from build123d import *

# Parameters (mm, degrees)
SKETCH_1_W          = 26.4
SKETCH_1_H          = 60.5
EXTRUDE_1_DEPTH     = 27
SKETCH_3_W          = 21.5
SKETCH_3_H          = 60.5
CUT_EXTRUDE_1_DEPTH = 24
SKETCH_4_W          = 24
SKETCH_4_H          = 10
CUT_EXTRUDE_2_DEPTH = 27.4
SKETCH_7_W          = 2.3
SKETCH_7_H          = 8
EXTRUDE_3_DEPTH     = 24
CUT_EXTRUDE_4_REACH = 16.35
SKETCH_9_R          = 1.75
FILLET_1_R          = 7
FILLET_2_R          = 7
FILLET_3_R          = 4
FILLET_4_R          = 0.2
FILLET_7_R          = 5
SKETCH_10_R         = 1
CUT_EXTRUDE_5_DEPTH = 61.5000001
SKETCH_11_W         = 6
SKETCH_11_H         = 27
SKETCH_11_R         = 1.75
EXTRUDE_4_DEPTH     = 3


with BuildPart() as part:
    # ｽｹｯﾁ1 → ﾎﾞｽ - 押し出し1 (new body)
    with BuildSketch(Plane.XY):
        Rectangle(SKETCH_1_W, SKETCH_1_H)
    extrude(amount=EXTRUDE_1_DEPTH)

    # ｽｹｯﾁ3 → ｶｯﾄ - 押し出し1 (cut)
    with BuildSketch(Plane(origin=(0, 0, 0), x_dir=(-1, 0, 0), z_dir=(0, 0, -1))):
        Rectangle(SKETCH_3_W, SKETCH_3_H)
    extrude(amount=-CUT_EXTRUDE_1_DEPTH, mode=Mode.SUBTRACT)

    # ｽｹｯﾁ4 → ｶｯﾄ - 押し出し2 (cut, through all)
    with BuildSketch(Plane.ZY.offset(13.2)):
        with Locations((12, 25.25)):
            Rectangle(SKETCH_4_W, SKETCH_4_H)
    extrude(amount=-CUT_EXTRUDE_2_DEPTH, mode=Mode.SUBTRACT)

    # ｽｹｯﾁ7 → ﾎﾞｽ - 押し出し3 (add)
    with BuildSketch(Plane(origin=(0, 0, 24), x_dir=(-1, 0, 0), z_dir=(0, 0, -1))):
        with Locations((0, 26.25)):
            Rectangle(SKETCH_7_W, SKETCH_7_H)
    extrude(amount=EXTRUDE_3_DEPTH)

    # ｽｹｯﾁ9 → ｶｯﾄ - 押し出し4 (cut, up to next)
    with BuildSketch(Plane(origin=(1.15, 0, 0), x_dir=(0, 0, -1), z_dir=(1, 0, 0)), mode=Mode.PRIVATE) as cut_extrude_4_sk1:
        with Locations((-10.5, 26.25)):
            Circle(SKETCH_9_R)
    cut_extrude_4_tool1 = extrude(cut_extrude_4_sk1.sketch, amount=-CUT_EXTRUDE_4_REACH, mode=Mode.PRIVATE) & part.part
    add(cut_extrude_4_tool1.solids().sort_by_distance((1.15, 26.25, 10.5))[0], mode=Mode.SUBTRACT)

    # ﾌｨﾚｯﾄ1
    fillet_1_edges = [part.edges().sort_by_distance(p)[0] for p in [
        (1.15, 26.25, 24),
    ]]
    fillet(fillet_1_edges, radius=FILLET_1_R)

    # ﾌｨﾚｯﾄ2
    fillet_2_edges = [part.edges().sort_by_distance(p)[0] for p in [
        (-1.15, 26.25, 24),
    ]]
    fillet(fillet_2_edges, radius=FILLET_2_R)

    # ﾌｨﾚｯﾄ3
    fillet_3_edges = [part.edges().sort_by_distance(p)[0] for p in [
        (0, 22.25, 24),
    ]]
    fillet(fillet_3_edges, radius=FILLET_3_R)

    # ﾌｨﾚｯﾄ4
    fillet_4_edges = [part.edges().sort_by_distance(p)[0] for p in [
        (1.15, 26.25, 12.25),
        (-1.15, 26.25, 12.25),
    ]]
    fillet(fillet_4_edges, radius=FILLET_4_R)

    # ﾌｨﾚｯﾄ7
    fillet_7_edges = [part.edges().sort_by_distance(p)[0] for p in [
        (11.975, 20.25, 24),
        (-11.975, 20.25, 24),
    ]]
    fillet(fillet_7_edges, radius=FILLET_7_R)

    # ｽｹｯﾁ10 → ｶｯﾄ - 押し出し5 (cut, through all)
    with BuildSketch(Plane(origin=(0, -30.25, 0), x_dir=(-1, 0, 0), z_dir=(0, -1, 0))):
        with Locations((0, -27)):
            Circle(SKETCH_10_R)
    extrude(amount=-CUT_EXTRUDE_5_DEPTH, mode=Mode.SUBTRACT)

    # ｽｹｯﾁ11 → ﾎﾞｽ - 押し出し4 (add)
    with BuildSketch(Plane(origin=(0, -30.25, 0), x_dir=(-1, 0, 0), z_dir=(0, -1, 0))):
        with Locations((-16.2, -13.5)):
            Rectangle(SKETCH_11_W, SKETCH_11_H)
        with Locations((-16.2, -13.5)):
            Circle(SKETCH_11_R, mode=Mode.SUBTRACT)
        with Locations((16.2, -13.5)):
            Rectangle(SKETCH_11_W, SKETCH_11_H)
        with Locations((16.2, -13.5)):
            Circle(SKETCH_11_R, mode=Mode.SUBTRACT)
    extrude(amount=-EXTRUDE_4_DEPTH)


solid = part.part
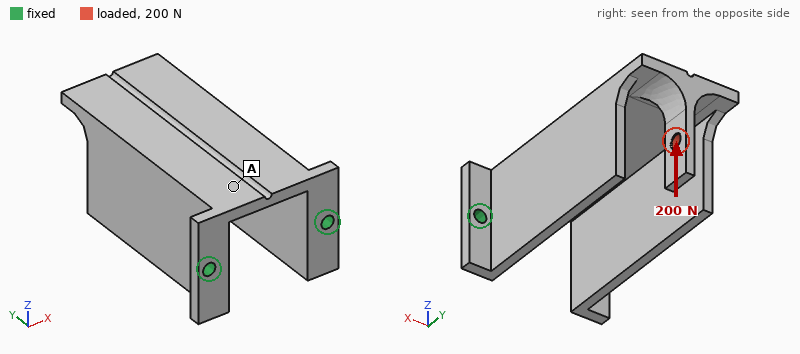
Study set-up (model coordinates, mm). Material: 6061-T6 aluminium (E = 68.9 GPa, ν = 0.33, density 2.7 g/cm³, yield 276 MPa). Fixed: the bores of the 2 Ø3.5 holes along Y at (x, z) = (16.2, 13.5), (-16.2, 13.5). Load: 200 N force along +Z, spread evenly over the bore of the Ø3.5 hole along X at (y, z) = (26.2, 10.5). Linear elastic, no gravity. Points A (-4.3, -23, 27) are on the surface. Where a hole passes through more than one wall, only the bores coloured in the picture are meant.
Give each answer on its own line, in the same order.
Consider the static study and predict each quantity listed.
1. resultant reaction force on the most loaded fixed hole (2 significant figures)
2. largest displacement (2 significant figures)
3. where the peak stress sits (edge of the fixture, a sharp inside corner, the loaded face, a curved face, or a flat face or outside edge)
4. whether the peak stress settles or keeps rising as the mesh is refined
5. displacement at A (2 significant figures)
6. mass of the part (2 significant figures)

100 N
0.36 mm
edge of the fixture
keeps rising
0.074 mm
33 g
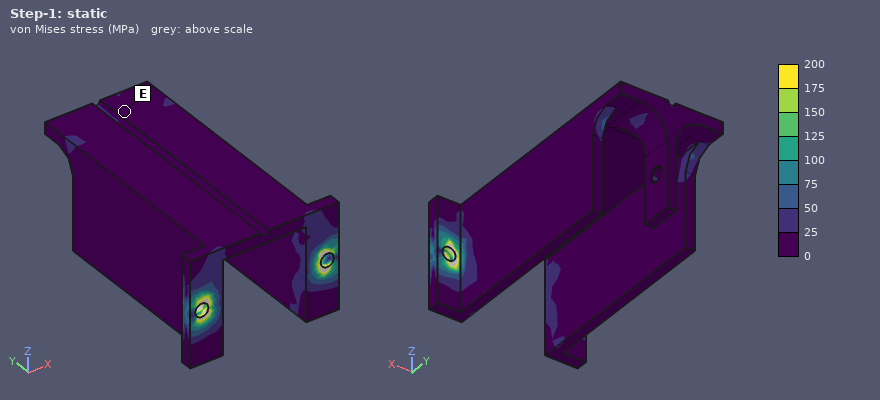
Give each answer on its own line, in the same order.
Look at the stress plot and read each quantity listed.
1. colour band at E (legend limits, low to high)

0 to 25 MPa
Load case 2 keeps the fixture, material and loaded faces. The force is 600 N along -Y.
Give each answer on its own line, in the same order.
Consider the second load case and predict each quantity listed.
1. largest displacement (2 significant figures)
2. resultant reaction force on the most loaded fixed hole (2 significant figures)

0.51 mm
300 N
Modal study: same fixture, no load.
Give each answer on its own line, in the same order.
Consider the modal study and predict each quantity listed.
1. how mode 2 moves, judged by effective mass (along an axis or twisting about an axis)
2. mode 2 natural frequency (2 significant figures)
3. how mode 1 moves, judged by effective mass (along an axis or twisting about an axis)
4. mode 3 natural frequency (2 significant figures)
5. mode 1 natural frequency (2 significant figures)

along X
1400 Hz
along Z
3300 Hz
1200 Hz
